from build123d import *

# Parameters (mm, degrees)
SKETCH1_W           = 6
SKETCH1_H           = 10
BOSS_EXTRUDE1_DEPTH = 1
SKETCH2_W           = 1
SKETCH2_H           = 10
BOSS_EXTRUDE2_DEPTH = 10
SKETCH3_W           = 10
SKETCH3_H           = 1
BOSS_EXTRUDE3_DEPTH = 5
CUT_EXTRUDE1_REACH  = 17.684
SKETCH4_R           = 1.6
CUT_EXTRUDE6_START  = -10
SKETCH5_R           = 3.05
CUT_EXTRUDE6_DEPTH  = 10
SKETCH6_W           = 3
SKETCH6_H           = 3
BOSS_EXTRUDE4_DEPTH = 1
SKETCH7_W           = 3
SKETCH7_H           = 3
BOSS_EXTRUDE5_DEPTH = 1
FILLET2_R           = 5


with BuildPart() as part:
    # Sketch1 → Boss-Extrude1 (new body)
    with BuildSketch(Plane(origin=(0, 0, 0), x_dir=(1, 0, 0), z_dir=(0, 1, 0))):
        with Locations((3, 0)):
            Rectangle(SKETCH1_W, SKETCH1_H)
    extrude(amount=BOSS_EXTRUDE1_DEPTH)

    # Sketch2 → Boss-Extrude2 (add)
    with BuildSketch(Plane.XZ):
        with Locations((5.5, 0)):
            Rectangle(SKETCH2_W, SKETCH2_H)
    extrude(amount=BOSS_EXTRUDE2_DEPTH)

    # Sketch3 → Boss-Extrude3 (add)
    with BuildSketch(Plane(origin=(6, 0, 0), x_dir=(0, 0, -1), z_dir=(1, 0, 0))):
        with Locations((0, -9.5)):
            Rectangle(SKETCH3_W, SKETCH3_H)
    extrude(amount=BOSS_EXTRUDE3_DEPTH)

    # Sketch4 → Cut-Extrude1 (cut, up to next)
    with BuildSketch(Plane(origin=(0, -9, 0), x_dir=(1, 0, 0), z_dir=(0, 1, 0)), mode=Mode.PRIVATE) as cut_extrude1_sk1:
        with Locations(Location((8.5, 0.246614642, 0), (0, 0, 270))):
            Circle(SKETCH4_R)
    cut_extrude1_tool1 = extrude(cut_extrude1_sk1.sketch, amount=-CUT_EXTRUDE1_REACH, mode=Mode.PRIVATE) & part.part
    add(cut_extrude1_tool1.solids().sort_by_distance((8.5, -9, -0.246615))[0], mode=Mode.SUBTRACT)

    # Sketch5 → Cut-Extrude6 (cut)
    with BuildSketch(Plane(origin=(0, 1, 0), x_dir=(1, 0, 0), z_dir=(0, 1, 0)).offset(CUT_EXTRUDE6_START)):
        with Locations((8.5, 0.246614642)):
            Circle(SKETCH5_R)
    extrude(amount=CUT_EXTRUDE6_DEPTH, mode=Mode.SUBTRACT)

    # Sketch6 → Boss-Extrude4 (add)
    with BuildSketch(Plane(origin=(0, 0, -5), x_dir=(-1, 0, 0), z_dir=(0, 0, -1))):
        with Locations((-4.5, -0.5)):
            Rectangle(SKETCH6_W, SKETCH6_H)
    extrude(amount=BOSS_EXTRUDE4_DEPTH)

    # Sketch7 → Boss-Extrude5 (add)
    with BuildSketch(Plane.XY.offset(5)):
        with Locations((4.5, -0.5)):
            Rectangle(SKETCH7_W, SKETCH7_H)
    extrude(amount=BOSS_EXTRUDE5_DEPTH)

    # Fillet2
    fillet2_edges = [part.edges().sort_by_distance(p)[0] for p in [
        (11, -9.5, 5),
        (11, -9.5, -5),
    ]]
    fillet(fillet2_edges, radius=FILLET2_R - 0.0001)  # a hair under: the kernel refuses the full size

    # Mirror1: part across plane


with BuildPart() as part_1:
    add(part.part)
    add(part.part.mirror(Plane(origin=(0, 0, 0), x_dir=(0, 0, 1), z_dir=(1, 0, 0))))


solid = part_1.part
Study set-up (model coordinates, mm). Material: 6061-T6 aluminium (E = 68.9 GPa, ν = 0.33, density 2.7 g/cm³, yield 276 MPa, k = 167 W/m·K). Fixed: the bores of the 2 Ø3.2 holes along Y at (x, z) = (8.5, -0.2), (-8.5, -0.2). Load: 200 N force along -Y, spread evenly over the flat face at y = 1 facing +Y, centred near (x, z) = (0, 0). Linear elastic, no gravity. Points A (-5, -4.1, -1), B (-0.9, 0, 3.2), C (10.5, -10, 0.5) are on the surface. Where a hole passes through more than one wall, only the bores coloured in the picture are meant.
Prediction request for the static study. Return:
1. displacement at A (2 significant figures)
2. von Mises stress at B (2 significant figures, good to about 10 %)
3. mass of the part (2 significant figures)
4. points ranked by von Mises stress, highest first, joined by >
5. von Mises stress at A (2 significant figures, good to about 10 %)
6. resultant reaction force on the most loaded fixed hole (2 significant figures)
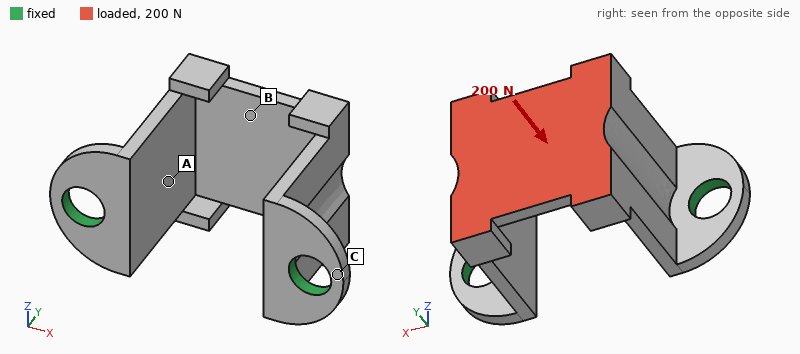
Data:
7.1 µm
55 MPa
1.1 g
B > A > C
29 MPa
100 N
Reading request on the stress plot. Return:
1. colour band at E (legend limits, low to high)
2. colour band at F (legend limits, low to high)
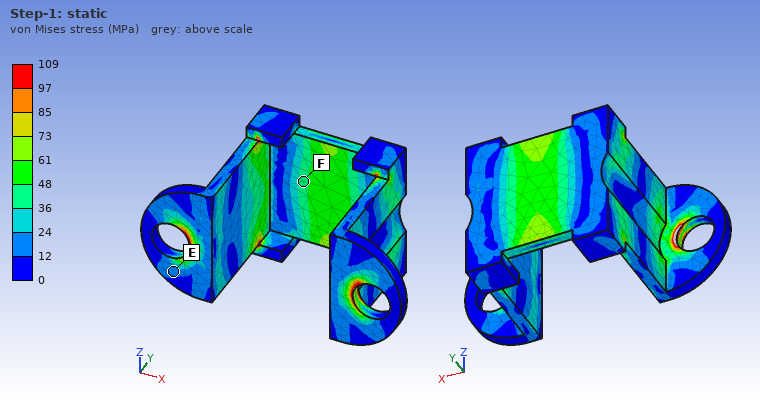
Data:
12 to 24 MPa
36 to 48 MPa
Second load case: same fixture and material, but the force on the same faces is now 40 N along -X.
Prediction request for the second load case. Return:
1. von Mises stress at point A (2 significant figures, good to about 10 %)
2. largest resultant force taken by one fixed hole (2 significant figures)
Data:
8.9 MPa
29 N
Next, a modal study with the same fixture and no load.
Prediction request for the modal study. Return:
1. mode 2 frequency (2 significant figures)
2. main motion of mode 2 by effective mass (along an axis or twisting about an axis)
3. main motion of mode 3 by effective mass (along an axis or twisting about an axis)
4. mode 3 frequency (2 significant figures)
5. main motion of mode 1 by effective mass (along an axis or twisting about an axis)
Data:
7300 Hz
along Z
twisting about Y
9400 Hz
along X
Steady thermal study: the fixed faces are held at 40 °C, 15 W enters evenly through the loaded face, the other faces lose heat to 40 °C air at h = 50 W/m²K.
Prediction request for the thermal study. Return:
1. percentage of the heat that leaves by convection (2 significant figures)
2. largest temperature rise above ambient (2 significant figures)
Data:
9.0 %
64 K
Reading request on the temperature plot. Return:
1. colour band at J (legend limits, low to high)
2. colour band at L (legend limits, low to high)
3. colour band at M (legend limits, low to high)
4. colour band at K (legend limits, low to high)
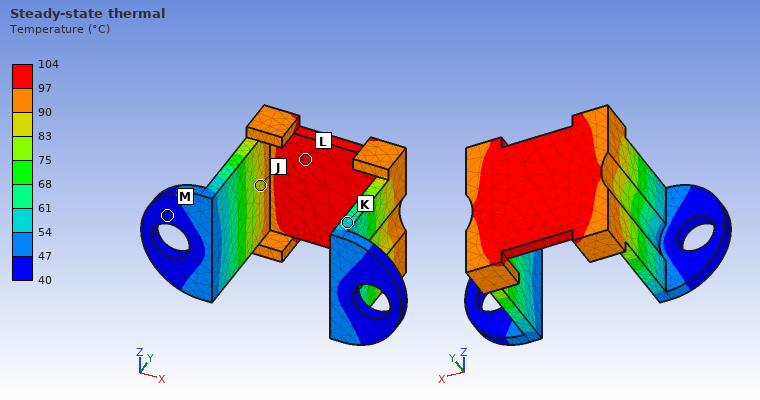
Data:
83 to 90 °C
97 to 104 °C
40 to 47 °C
54 to 61 °C
